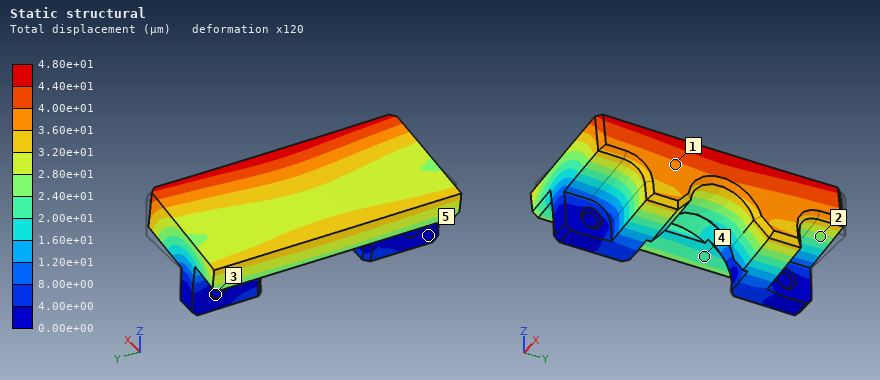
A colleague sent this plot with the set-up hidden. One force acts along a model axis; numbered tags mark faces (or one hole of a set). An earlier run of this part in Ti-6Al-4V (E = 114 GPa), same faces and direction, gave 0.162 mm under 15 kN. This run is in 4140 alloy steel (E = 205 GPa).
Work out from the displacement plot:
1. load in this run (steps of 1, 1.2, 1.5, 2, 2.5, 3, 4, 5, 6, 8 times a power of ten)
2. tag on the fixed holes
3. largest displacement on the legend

8 kN
3
4.80e+01 µm
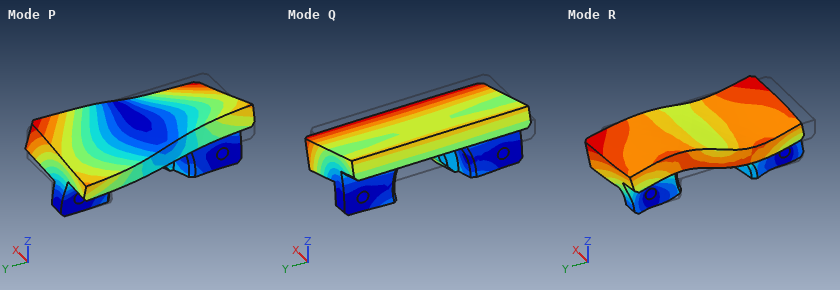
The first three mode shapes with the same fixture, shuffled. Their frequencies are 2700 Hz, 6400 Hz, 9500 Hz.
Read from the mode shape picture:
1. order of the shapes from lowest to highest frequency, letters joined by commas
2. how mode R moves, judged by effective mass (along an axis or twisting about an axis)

Q, P, R
along Y
